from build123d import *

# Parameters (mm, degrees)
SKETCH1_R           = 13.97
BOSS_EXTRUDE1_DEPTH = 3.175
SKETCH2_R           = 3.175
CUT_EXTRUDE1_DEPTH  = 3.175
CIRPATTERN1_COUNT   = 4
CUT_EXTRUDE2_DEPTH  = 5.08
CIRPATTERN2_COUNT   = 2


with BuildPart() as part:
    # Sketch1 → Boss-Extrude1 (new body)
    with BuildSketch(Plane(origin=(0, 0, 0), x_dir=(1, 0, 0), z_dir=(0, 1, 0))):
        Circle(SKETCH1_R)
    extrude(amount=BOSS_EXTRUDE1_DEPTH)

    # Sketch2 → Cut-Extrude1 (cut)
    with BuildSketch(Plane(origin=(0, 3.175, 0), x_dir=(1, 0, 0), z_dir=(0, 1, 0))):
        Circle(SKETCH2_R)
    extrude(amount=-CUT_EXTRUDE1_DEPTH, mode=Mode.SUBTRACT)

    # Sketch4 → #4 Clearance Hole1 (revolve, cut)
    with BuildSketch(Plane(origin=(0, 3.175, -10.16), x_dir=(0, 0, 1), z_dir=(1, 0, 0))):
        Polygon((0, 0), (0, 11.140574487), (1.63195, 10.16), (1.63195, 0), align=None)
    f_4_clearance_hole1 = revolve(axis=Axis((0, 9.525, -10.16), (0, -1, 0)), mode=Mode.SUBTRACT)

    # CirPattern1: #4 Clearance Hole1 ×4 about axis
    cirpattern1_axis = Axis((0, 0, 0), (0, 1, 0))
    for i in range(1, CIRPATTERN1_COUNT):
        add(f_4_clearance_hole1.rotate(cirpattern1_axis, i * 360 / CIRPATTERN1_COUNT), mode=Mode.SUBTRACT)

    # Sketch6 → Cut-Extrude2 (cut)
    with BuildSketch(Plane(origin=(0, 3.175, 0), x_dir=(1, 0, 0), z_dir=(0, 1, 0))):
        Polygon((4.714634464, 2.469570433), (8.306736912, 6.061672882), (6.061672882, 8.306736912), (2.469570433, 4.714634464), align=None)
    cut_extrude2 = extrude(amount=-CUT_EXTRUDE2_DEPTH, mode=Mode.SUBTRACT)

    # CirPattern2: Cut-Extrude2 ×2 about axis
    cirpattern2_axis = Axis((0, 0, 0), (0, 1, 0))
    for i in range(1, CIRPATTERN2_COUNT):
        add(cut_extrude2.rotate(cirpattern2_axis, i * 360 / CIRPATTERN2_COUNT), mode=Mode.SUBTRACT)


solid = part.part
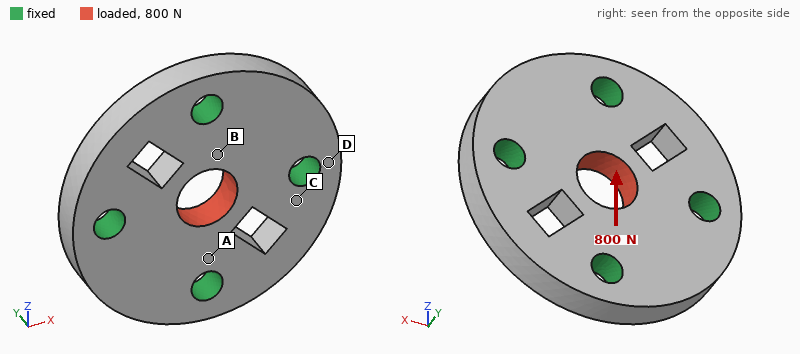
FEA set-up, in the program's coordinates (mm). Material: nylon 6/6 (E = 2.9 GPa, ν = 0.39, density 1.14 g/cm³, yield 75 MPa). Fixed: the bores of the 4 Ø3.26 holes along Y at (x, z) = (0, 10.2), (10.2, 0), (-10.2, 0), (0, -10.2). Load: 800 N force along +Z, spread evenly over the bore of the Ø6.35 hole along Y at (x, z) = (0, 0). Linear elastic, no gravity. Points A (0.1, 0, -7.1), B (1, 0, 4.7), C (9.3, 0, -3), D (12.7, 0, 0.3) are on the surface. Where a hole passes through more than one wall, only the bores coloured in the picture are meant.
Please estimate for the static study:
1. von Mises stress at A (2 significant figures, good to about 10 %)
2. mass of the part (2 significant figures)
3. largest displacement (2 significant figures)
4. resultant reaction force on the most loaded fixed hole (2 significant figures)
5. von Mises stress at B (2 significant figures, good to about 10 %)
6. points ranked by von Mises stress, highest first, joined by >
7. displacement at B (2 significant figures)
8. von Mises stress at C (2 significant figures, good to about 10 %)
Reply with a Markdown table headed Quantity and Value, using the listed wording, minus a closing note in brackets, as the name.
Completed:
| Quantity | Value |
|---|---|
| von Mises stress at A | 17 MPa |
| mass of the part | 1.9 g |
| largest displacement | 45 µm |
| resultant reaction force on the most loaded fixed hole | 270 N |
| von Mises stress at B | 14 MPa |
| points ranked by von Mises stress, highest first, joined by > | A > B > C > D |
| displacement at B | 22 µm |
| von Mises stress at C | 4.8 MPa |
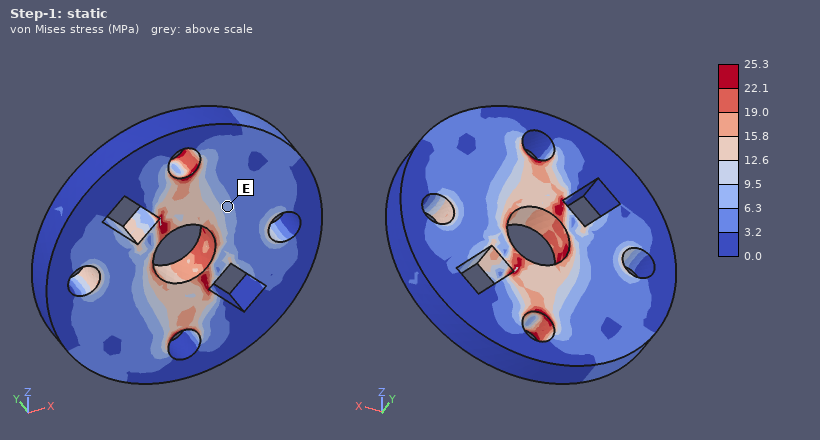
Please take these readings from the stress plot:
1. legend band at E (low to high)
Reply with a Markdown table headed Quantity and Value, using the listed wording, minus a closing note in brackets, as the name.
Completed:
| Quantity | Value |
|---|---|
| legend band at E | 6.3 to 9.5 MPa |
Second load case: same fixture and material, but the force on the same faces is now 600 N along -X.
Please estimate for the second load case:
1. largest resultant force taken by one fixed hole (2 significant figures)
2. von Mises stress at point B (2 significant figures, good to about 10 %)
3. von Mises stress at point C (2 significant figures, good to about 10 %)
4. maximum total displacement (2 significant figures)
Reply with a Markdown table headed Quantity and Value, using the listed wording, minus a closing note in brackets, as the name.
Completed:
| Quantity | Value |
|---|---|
| largest resultant force taken by one fixed hole | 200 N |
| von Mises stress at point B | 5.6 MPa |
| von Mises stress at point C | 4.2 MPa |
| maximum total displacement | 33 µm |
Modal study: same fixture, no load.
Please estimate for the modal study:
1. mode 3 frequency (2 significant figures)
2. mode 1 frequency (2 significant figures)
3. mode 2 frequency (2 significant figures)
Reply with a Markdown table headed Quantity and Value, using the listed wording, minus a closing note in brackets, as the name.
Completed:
| Quantity | Value |
|---|---|
| mode 3 frequency | 17 kHz |
| mode 1 frequency | 16 kHz |
| mode 2 frequency | 17 kHz |
